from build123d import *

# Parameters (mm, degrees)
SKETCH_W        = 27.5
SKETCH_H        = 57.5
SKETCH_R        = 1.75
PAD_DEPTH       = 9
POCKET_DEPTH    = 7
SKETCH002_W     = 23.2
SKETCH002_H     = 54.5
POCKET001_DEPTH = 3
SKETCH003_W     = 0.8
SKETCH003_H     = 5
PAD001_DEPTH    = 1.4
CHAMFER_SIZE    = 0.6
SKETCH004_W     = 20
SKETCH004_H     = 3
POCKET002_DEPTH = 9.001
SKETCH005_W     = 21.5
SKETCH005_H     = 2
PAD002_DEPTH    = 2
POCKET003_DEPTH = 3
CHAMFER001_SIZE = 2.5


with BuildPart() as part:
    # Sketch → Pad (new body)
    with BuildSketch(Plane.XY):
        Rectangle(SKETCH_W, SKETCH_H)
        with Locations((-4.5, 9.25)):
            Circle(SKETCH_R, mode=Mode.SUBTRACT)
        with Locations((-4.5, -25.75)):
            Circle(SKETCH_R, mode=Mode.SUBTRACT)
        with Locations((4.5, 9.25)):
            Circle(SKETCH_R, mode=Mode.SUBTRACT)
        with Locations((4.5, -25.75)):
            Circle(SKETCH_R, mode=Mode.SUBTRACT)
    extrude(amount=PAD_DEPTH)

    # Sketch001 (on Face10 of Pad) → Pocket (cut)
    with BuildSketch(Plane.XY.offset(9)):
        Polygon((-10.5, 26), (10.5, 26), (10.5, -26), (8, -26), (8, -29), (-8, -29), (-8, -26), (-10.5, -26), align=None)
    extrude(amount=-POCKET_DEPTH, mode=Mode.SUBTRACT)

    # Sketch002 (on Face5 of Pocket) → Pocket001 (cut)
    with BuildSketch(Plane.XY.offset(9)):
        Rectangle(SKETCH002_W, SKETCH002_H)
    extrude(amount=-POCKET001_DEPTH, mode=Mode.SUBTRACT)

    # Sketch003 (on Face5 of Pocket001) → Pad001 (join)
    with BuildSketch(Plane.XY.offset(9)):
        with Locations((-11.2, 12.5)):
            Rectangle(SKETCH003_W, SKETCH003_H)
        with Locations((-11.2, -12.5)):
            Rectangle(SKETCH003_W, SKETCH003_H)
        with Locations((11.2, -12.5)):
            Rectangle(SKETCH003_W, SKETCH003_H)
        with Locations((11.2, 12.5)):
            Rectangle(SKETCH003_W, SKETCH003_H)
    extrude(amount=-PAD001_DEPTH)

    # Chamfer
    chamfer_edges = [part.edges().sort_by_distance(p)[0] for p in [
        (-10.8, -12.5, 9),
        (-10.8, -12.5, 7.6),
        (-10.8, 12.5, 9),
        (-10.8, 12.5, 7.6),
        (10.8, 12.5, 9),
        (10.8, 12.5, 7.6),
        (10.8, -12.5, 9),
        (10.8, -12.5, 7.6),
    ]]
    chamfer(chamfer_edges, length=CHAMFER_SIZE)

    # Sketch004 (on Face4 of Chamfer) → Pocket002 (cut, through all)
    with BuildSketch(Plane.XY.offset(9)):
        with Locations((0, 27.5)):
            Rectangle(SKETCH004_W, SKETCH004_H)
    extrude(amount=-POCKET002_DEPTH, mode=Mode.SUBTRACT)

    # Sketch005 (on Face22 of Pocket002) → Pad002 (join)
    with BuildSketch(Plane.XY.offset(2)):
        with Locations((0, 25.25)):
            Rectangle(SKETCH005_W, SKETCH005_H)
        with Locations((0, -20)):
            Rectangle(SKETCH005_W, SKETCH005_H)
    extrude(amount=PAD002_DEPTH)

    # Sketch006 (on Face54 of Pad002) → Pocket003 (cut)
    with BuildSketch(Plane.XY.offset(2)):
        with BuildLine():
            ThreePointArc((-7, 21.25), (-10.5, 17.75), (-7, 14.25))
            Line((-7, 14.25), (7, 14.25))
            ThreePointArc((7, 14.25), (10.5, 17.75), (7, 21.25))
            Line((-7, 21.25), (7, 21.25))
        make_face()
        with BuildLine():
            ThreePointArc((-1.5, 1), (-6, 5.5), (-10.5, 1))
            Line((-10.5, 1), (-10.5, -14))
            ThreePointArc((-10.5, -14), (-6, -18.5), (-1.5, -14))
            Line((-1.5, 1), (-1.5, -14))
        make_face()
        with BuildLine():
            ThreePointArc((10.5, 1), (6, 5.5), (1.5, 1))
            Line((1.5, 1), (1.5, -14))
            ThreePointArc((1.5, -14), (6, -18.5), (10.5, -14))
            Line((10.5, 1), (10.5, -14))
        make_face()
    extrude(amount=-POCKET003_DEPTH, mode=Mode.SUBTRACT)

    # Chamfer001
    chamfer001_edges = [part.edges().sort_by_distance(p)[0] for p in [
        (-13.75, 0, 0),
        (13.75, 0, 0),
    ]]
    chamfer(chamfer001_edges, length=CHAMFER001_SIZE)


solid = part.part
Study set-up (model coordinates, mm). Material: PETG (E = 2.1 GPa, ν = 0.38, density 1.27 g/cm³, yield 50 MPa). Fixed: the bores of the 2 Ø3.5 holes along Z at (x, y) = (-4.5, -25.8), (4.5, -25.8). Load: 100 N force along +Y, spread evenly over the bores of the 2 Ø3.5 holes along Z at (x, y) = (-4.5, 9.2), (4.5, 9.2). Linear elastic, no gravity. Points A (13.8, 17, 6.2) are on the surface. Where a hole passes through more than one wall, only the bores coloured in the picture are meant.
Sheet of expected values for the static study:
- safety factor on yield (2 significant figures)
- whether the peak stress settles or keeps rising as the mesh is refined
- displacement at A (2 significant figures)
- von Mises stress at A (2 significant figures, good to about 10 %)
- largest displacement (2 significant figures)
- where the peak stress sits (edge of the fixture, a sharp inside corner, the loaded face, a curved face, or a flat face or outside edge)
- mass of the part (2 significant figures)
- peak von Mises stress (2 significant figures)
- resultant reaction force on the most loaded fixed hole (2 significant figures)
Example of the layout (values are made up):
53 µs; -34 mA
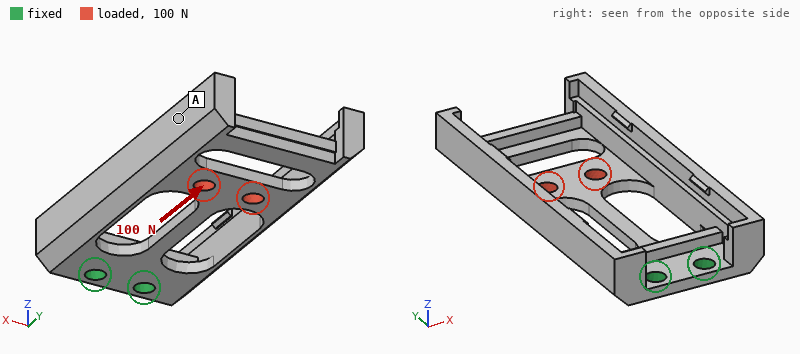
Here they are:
5.1; settles; 0.23 mm; 1.2 MPa; 0.37 mm; a curved face; 5.2 g; 9.9 MPa; 51 N
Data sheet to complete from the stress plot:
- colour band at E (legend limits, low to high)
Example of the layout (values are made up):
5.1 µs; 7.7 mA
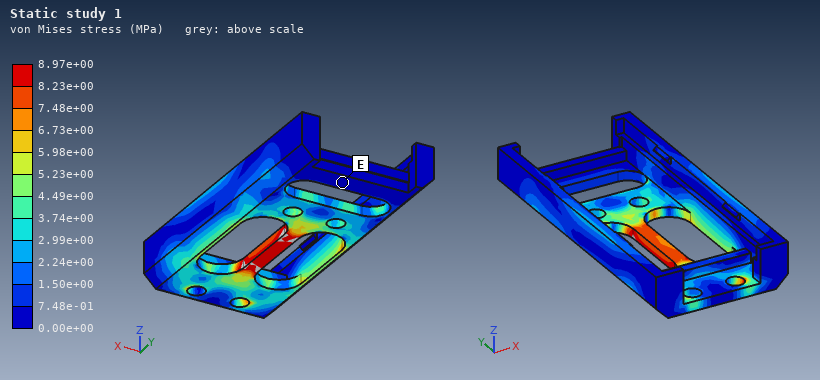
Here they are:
0.00e+00 to 7.48e-01 MPa
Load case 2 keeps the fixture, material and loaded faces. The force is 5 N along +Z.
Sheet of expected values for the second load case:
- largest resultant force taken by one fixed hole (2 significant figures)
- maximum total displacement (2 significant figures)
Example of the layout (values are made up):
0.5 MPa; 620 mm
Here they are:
3.3 N; 0.75 mm
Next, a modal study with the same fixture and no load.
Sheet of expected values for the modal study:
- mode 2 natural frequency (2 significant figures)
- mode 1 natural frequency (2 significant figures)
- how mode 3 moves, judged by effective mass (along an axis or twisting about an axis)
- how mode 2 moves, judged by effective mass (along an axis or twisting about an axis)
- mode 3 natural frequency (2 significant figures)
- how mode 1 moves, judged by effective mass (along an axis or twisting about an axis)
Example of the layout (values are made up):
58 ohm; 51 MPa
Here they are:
440 Hz; 260 Hz; along X; along X; 580 Hz; along Z
